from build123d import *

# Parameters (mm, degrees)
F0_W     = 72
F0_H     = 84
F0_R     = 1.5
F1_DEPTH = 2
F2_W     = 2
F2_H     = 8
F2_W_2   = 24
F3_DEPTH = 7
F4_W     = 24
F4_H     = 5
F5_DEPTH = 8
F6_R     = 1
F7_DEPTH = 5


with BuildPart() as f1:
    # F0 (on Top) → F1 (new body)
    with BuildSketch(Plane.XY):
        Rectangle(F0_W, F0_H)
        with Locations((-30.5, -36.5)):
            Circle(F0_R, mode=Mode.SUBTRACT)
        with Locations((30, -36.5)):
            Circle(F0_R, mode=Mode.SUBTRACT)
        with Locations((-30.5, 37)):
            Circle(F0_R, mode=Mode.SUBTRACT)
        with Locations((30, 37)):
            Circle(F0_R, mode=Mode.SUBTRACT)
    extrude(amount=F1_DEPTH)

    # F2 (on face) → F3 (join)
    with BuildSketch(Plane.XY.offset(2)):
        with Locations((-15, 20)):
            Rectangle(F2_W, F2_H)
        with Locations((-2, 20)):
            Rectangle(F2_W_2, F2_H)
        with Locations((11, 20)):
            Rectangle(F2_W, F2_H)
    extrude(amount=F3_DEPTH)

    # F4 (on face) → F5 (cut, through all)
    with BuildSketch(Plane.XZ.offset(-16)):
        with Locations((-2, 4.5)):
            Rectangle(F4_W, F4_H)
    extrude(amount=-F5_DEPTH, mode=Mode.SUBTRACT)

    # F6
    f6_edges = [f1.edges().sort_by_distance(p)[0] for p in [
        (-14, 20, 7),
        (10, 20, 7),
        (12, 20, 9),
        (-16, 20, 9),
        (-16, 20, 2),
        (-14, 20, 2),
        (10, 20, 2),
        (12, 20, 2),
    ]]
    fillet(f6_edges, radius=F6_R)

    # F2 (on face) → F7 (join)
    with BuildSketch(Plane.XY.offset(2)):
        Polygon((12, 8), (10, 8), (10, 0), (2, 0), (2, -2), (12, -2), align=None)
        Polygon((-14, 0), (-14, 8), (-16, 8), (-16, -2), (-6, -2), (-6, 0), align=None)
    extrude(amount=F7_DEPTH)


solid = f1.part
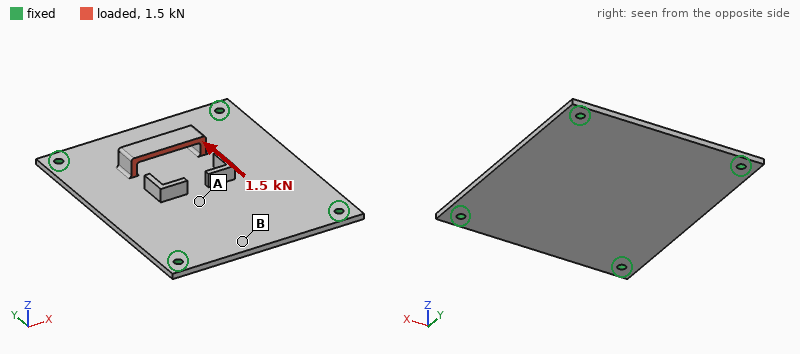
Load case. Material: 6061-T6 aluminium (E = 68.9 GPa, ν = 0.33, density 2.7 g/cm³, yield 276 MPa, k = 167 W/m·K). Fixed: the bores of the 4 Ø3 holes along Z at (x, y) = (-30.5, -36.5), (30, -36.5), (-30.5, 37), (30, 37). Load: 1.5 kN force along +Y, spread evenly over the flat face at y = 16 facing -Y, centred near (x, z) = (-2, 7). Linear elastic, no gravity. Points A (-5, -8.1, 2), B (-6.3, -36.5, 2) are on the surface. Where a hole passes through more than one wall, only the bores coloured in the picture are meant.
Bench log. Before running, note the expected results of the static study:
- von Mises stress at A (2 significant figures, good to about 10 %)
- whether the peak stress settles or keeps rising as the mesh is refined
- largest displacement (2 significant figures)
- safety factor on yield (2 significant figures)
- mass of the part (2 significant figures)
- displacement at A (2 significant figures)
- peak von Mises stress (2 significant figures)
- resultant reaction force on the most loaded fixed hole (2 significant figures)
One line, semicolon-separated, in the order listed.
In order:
38 MPa; settles; 0.31 mm; 0.45; 35 g; 0.25 mm; 610 MPa; 500 N
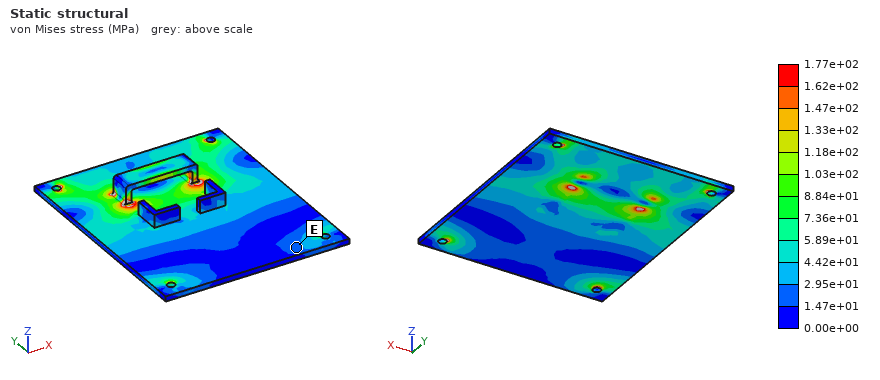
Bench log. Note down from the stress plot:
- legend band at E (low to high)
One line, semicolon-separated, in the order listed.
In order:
1.47e+01 to 2.95e+01 MPa
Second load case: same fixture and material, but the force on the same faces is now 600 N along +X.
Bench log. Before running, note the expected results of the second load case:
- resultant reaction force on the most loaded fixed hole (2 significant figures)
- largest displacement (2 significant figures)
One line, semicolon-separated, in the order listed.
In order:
250 N; 69 µm
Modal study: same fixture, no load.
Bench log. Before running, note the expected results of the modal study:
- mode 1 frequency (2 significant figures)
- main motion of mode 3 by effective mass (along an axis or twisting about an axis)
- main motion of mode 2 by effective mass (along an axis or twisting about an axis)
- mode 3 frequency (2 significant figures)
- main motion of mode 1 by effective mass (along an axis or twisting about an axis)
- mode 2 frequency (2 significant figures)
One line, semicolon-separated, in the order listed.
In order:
1400 Hz; twisting about X; twisting about Y; 2900 Hz; along Z; 2300 Hz
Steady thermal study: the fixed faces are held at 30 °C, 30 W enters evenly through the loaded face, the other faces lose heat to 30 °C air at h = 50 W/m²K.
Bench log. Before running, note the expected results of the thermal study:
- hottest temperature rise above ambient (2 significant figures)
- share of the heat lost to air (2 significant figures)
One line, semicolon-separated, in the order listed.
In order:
81 K; 33 %
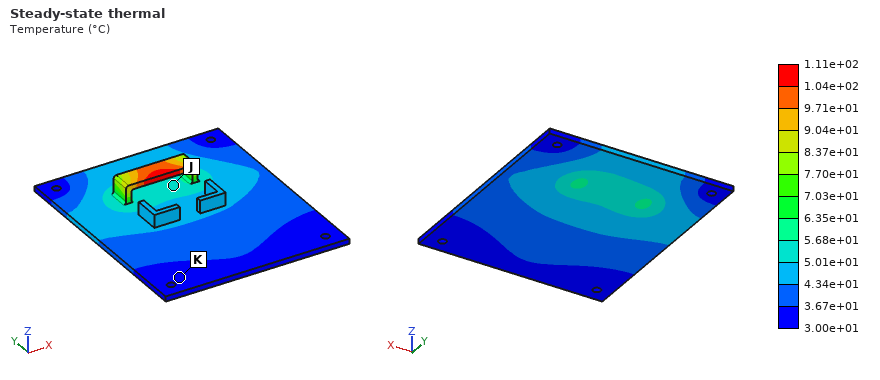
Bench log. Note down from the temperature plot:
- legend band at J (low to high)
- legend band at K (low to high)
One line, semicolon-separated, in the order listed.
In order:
5.01e+01 to 5.68e+01 °C; 3.00e+01 to 3.67e+01 °C
